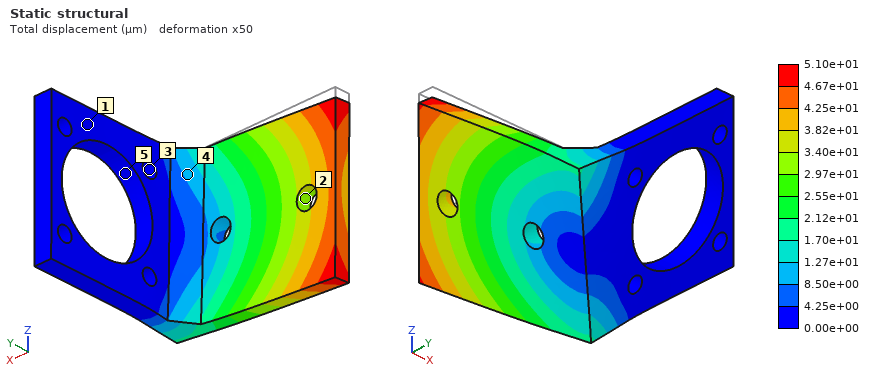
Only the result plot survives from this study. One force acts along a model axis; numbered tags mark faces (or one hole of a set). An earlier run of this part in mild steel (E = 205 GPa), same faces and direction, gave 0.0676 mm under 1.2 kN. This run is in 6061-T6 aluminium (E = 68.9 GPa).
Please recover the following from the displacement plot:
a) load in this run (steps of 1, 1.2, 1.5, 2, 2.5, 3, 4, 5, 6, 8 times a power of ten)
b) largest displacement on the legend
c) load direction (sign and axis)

300 N
5.10e+01 µm
-Z
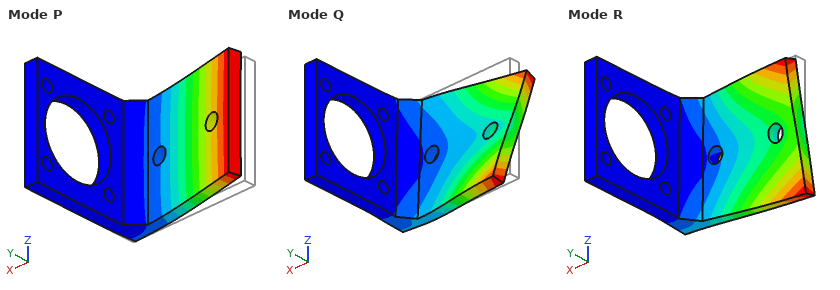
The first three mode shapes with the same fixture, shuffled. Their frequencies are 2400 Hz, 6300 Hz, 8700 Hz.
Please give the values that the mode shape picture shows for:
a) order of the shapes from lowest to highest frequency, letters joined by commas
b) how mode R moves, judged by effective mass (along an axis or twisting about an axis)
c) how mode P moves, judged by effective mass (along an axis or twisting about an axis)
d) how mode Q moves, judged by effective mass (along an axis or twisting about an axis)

P, R, Q
along Z
along Y
along Z
